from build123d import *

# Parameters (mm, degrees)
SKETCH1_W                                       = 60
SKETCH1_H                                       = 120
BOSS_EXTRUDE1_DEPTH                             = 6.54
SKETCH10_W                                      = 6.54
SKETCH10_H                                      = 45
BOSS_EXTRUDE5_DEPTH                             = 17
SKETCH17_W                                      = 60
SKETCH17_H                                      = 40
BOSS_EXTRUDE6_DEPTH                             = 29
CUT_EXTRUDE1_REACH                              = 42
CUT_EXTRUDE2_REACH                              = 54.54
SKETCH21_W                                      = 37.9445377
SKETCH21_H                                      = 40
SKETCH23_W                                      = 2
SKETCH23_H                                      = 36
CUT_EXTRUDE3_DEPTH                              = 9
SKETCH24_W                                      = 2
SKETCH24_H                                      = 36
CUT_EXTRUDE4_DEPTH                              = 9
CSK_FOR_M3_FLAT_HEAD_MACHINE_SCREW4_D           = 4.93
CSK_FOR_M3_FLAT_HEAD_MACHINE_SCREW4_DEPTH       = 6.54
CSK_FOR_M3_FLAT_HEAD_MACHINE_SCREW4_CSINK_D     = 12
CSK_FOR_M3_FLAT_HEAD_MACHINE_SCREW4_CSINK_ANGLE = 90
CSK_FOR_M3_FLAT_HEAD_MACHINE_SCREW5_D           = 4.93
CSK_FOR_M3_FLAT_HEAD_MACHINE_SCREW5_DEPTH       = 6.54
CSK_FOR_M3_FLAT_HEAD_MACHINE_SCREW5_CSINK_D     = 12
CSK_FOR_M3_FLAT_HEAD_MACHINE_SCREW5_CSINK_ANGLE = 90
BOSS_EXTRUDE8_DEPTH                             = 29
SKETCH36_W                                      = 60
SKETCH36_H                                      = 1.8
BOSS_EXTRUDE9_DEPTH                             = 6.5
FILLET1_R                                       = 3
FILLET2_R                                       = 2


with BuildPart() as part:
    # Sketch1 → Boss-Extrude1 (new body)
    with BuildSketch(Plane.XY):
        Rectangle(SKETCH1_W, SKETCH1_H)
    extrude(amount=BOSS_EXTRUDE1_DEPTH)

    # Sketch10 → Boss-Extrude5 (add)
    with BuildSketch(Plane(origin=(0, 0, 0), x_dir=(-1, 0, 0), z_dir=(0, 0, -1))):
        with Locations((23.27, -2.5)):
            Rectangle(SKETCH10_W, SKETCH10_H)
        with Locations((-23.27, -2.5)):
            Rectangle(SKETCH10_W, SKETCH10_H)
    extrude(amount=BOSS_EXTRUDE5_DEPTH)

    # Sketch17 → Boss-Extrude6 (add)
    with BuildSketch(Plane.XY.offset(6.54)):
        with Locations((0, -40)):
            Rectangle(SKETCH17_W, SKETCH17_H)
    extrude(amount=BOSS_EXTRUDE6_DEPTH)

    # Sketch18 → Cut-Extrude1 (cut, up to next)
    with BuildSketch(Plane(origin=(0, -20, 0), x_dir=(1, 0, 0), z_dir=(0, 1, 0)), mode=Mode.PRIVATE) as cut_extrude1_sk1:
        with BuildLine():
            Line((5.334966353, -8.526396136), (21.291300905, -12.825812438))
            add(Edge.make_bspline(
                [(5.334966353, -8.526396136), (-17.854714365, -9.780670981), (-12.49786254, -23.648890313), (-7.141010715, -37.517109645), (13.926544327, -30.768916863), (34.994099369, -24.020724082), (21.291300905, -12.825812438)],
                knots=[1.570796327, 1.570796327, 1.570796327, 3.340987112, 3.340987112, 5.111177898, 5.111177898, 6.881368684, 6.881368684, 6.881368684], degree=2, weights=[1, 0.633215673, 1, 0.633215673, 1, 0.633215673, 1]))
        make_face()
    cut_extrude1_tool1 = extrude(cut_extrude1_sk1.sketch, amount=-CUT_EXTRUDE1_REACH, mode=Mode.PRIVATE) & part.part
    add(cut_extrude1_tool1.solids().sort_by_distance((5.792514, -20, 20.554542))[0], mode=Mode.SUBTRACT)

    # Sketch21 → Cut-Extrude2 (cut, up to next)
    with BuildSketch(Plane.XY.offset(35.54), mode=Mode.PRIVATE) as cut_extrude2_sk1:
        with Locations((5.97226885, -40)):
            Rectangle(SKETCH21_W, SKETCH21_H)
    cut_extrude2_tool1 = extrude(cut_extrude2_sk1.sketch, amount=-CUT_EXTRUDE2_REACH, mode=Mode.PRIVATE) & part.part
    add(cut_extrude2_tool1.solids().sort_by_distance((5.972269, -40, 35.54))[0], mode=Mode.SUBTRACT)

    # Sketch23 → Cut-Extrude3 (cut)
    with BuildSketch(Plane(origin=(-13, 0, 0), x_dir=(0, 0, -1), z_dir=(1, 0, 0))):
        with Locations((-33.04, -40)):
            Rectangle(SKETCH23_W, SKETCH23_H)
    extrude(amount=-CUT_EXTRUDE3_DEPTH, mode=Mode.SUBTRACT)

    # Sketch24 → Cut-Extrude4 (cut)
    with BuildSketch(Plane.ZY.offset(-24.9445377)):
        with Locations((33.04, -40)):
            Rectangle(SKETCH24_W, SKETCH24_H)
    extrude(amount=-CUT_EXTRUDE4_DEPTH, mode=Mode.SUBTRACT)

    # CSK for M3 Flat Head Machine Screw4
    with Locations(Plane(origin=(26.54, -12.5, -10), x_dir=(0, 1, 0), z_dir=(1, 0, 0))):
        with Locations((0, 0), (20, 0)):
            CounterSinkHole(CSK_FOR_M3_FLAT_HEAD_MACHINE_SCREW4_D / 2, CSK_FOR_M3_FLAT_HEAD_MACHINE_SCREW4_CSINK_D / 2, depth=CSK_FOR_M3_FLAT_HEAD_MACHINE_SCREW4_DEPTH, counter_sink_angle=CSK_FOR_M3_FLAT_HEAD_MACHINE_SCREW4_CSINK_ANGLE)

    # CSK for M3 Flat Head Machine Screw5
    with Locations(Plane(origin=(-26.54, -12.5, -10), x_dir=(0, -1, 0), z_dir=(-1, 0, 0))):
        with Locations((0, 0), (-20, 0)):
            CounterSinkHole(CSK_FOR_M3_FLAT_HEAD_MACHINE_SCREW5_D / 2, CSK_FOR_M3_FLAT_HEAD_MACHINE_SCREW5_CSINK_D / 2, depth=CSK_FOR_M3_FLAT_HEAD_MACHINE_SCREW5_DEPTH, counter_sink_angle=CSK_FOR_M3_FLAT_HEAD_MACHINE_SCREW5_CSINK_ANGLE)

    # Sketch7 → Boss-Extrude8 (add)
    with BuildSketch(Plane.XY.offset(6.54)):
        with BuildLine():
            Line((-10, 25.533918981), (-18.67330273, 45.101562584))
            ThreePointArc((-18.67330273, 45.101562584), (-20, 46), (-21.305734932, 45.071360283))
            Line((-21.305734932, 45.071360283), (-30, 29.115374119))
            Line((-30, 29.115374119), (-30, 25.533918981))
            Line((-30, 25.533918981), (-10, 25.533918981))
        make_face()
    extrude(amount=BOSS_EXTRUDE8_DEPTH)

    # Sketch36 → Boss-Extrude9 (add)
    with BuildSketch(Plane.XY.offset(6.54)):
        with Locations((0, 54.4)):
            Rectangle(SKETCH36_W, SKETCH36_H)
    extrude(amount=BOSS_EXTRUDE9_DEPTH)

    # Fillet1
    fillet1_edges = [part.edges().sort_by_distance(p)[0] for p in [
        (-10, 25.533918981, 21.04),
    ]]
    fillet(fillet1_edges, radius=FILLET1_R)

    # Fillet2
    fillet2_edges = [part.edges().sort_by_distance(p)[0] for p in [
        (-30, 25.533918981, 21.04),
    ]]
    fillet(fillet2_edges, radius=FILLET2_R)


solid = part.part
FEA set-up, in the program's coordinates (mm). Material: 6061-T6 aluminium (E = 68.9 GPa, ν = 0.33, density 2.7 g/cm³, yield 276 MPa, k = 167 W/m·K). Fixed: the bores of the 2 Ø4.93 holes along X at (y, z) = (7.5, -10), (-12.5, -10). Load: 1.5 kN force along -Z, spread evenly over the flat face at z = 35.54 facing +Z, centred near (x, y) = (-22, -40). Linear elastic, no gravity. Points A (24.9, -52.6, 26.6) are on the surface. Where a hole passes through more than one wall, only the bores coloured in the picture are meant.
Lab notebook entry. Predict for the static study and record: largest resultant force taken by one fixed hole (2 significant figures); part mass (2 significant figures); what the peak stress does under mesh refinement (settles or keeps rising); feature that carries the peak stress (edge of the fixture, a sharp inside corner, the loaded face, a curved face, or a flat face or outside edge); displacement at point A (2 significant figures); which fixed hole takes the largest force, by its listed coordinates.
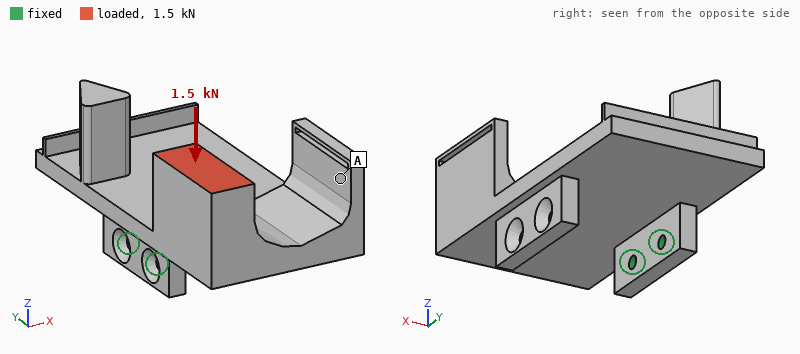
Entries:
3.2 kN
260 g
keeps rising
edge of the fixture
0.19 mm
(-12.5, -10)
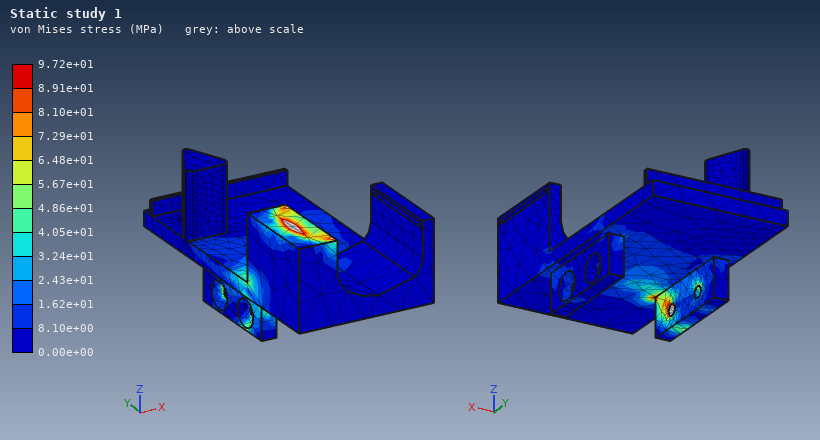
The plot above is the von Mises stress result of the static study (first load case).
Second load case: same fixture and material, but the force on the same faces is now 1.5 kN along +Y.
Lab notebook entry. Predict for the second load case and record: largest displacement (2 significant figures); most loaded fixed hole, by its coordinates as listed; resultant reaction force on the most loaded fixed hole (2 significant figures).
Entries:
0.33 mm
(7.5, -10)
3.2 kN
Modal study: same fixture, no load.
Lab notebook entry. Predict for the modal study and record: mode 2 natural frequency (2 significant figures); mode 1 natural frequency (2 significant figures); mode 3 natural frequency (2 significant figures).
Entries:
880 Hz
510 Hz
1100 Hz
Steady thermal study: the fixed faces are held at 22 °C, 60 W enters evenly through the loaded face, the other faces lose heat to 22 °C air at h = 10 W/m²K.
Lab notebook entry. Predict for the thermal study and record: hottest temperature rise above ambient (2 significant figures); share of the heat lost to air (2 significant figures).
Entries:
71 K
12 %
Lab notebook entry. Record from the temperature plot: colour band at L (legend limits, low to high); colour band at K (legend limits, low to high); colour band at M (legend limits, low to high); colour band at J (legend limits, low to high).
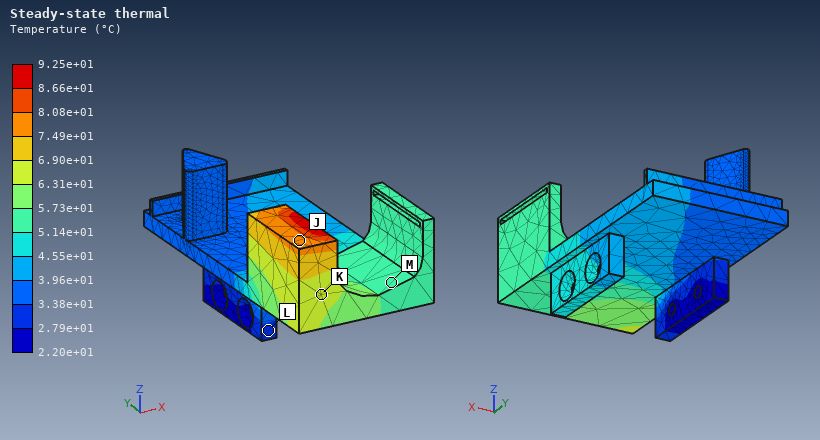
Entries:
2.79e+01 to 3.38e+01 °C
6.31e+01 to 6.90e+01 °C
5.14e+01 to 5.73e+01 °C
7.49e+01 to 8.08e+01 °C
